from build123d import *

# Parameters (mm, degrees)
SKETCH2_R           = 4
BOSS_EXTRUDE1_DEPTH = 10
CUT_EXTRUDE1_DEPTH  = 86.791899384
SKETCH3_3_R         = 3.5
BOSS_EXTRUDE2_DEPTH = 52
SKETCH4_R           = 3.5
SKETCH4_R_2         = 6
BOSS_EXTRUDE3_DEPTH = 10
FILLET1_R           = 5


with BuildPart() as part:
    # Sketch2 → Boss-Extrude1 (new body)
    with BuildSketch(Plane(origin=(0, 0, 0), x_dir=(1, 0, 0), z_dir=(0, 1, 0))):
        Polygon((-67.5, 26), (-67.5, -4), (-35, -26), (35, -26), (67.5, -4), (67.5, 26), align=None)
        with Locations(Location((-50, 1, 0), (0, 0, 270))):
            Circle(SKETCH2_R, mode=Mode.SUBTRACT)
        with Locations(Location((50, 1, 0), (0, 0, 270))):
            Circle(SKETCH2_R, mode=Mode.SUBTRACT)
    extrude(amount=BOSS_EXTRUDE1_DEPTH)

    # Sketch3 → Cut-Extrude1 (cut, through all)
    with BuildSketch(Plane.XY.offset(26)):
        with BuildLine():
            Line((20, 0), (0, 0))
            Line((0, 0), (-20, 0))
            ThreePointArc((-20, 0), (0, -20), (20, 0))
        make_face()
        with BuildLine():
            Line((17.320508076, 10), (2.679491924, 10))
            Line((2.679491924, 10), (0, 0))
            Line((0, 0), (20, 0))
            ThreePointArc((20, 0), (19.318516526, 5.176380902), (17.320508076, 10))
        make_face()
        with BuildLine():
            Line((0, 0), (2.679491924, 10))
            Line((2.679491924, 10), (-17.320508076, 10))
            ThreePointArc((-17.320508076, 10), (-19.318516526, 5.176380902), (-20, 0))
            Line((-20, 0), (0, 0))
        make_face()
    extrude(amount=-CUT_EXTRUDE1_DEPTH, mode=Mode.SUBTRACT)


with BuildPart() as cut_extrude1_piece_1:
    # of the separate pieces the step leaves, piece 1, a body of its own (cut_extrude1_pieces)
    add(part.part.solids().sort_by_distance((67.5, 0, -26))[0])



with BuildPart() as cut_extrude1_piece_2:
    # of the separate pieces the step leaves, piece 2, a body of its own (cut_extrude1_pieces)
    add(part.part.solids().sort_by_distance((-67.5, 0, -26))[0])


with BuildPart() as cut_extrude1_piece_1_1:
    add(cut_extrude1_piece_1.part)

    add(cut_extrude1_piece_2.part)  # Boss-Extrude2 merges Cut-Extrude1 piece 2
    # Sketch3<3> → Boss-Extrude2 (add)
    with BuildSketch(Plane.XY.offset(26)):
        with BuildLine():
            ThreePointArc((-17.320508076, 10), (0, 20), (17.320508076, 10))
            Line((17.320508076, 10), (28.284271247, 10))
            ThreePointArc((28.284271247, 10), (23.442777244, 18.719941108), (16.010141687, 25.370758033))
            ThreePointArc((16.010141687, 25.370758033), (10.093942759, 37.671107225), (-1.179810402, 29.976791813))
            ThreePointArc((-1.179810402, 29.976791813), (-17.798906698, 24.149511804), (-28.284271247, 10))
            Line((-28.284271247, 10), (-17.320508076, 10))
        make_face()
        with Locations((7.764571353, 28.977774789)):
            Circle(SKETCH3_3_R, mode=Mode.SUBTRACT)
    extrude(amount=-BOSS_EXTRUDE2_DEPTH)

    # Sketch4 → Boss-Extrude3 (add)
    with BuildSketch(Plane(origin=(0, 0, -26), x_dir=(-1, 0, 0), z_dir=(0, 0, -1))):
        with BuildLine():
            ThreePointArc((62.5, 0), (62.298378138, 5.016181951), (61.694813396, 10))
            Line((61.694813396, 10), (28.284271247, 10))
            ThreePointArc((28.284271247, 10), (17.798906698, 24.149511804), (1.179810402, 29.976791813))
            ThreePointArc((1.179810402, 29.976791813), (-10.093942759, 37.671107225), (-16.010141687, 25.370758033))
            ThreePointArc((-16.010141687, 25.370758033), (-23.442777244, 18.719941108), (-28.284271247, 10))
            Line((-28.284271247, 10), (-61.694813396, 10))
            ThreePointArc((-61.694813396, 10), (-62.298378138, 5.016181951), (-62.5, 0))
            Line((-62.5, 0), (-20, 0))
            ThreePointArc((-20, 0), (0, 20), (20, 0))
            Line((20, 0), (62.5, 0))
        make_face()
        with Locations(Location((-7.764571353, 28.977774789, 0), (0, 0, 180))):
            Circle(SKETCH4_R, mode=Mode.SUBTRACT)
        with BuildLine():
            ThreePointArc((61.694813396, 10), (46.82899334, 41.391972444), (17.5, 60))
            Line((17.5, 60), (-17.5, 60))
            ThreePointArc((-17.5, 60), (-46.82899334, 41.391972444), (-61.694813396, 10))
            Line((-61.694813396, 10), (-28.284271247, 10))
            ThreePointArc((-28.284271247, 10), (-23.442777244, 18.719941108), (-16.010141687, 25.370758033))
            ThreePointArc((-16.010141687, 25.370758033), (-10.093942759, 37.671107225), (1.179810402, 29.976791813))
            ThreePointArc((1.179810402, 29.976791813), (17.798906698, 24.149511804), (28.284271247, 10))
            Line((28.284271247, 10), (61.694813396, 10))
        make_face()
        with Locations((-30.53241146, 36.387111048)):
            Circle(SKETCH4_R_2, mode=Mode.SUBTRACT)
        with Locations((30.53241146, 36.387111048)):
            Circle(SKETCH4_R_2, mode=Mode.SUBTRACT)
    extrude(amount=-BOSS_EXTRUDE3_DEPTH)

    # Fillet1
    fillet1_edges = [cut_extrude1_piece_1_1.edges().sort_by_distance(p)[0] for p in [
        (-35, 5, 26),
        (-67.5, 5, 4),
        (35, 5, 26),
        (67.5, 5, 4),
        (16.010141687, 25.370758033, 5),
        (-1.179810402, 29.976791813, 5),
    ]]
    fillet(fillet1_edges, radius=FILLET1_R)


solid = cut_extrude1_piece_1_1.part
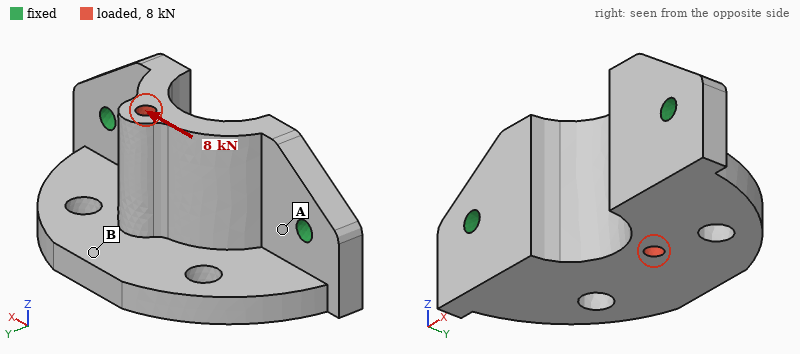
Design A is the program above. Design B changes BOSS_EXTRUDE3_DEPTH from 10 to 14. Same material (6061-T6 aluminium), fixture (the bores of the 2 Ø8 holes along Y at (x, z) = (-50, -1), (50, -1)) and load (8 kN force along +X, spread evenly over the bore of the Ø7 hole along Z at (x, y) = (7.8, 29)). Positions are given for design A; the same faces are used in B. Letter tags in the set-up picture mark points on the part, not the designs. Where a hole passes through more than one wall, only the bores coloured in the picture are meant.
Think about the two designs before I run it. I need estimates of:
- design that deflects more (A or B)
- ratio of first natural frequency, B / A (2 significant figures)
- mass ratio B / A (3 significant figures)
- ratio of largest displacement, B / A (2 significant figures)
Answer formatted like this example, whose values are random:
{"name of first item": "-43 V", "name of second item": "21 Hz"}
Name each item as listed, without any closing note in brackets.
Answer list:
{"design that deflects more": "A", "ratio of first natural frequency, B / A": "0.94", "mass ratio B / A": "1.13", "ratio of largest displacement, B / A": "0.92"}
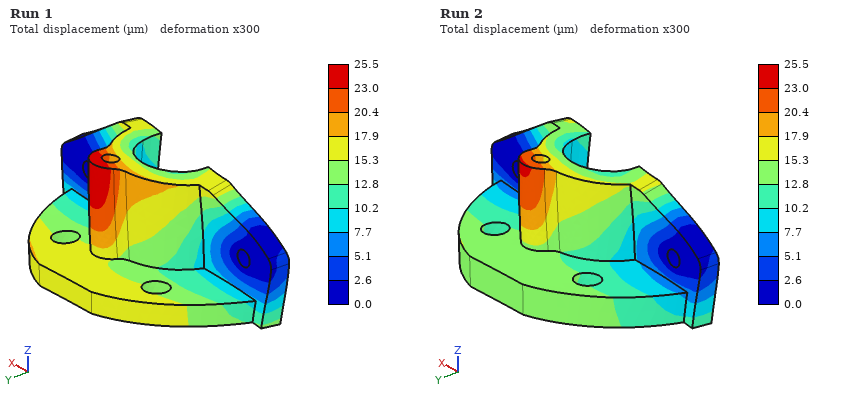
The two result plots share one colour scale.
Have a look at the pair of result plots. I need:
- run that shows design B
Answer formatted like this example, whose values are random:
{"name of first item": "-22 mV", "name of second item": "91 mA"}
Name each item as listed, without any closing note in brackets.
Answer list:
{"run that shows design B": "Run 2"}
